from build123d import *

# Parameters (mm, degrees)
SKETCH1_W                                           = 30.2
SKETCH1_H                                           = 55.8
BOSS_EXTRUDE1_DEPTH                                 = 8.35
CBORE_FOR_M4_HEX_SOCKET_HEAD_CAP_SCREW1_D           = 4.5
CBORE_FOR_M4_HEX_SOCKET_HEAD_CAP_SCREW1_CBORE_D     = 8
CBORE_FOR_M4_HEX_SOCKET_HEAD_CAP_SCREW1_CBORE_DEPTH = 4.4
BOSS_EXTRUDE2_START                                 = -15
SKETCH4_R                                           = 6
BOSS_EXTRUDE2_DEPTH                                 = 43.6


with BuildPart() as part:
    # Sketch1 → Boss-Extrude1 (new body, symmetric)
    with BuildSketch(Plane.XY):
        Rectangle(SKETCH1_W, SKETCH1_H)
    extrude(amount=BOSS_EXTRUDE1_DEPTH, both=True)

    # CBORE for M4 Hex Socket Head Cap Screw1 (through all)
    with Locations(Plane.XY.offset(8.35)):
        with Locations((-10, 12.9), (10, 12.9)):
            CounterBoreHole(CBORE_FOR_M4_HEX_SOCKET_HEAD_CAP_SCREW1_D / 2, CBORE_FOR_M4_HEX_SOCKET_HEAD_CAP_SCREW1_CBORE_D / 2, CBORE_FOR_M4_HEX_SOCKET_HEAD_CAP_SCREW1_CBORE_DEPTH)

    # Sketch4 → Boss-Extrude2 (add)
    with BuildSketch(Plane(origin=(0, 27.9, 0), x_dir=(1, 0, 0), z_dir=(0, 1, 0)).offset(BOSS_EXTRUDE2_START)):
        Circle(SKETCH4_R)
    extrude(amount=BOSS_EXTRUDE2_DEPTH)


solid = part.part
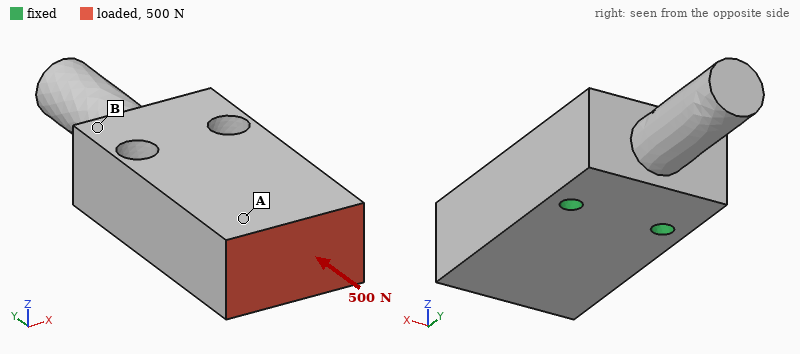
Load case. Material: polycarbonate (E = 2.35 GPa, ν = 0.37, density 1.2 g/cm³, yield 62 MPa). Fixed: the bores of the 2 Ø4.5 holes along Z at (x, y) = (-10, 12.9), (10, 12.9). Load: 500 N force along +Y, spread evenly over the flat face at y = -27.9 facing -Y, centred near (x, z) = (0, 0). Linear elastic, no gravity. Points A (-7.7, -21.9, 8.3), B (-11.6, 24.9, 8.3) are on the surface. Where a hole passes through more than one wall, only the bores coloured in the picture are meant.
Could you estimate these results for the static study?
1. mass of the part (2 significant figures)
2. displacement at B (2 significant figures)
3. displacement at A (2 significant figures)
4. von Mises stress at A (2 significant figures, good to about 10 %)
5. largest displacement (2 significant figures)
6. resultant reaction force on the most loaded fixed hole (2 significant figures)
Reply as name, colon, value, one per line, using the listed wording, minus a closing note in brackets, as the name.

mass of the part: 37 g
displacement at B: 5.6 µm
displacement at A: 27 µm
von Mises stress at A: 0.99 MPa
largest displacement: 31 µm
resultant reaction force on the most loaded fixed hole: 250 N
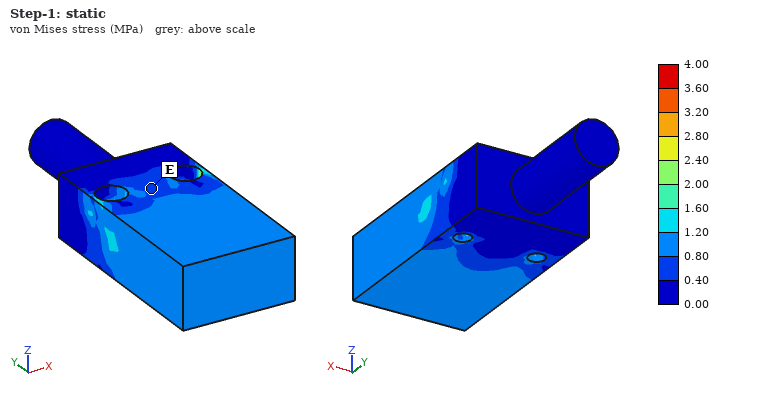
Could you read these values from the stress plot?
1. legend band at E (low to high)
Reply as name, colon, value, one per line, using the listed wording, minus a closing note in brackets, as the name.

legend band at E: 0.40 to 0.80 MPa
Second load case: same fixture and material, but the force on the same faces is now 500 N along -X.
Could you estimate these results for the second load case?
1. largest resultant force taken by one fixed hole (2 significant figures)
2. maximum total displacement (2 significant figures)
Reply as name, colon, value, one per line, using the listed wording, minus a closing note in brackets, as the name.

largest resultant force taken by one fixed hole: 960 N
maximum total displacement: 0.22 mm
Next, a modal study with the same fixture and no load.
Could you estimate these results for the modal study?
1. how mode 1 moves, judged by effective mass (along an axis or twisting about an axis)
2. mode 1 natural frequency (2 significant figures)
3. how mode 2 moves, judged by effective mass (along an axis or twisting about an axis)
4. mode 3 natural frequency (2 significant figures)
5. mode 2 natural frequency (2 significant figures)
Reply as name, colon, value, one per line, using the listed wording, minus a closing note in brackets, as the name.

how mode 1 moves, judged by effective mass: along Z
mode 1 natural frequency: 1600 Hz
how mode 2 moves, judged by effective mass: along Z
mode 3 natural frequency: 2200 Hz
mode 2 natural frequency: 2000 Hz
